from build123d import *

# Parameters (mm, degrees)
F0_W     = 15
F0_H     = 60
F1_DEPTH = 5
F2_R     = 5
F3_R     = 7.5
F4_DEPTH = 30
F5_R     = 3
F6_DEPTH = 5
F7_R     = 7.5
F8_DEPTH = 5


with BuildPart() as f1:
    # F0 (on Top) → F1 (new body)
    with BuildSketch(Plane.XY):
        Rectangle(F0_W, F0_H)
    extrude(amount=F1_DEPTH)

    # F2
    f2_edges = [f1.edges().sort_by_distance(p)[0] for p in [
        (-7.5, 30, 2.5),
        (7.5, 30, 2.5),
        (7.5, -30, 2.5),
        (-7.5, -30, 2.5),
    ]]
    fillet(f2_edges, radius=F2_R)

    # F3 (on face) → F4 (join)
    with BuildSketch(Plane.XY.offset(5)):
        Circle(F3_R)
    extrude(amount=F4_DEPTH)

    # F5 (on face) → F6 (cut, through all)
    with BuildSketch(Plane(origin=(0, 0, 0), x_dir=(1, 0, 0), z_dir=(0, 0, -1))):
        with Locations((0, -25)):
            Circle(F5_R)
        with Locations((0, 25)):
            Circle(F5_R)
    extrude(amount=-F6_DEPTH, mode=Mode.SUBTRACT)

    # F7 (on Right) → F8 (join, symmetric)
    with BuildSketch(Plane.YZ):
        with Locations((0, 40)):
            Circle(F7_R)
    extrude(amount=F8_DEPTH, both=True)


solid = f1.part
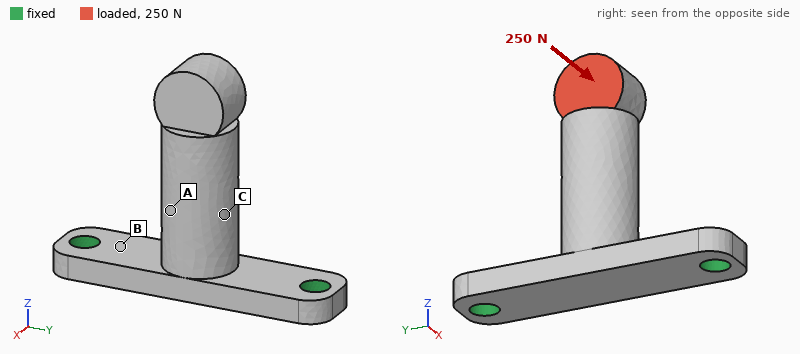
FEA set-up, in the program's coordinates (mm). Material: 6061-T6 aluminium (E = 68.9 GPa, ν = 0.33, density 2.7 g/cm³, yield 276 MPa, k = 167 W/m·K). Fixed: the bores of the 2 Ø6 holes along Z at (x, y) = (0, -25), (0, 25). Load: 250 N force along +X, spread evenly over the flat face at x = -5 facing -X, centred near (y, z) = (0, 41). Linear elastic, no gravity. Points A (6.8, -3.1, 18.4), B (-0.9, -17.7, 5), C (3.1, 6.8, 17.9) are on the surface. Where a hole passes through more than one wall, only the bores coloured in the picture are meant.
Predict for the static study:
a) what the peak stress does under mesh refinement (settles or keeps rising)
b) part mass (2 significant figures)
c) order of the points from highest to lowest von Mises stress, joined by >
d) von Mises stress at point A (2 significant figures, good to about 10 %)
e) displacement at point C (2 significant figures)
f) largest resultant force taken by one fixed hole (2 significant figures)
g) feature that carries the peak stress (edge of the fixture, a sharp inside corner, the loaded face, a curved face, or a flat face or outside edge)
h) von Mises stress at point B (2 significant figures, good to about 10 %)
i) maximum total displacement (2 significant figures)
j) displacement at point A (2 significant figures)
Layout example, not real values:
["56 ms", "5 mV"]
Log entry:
["keeps rising", "30 g", "B > A > C", "15 MPa", "0.10 mm", "130 N", "edge of the fixture", "71 MPa", "0.31 mm", "0.11 mm"]
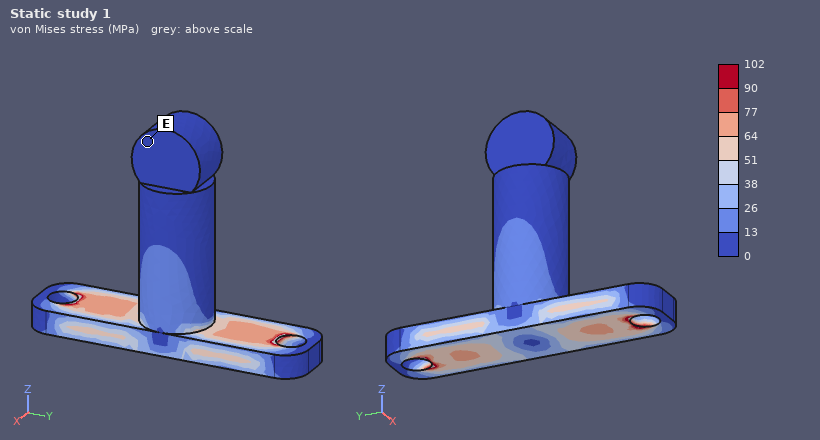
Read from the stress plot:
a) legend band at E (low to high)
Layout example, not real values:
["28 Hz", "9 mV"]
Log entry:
["0 to 13 MPa"]
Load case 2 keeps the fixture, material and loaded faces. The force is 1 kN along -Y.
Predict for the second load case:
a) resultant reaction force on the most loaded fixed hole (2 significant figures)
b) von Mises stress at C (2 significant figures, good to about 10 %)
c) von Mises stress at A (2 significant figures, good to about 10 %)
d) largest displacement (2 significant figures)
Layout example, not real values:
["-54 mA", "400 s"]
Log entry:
["1.3 kN", "63 MPa", "28 MPa", "0.36 mm"]
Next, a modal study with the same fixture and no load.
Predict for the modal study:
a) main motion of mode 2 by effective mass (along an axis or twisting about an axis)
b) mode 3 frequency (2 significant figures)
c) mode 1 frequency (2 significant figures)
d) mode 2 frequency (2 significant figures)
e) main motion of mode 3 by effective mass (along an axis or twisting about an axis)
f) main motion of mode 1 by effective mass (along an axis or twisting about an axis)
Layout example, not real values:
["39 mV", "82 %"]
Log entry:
["along Y", "5800 Hz", "1700 Hz", "3400 Hz", "along Z", "along X"]
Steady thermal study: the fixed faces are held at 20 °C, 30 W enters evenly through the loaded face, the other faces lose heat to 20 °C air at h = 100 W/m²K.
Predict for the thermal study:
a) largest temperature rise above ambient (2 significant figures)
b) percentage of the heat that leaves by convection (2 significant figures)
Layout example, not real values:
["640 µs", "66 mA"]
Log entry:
["54 K", "28 %"]
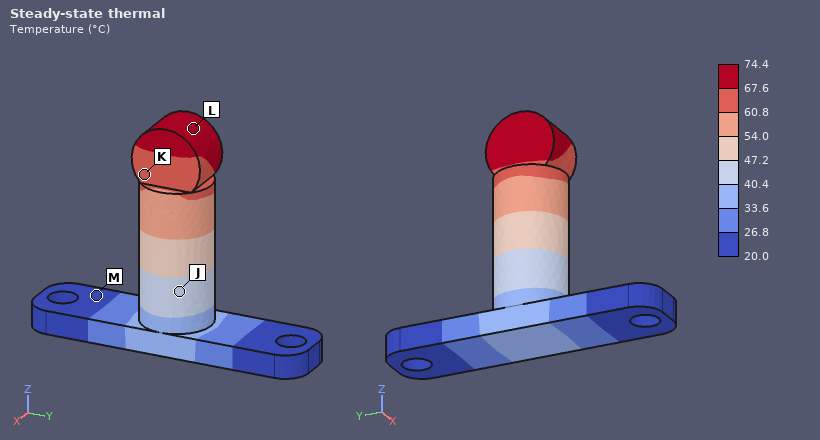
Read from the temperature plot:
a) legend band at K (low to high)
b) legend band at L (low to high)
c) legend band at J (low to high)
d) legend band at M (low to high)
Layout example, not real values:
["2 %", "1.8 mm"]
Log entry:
["60.8 to 67.6 °C", "67.6 to 74.4 °C", "40.4 to 47.2 °C", "20.0 to 26.8 °C"]
